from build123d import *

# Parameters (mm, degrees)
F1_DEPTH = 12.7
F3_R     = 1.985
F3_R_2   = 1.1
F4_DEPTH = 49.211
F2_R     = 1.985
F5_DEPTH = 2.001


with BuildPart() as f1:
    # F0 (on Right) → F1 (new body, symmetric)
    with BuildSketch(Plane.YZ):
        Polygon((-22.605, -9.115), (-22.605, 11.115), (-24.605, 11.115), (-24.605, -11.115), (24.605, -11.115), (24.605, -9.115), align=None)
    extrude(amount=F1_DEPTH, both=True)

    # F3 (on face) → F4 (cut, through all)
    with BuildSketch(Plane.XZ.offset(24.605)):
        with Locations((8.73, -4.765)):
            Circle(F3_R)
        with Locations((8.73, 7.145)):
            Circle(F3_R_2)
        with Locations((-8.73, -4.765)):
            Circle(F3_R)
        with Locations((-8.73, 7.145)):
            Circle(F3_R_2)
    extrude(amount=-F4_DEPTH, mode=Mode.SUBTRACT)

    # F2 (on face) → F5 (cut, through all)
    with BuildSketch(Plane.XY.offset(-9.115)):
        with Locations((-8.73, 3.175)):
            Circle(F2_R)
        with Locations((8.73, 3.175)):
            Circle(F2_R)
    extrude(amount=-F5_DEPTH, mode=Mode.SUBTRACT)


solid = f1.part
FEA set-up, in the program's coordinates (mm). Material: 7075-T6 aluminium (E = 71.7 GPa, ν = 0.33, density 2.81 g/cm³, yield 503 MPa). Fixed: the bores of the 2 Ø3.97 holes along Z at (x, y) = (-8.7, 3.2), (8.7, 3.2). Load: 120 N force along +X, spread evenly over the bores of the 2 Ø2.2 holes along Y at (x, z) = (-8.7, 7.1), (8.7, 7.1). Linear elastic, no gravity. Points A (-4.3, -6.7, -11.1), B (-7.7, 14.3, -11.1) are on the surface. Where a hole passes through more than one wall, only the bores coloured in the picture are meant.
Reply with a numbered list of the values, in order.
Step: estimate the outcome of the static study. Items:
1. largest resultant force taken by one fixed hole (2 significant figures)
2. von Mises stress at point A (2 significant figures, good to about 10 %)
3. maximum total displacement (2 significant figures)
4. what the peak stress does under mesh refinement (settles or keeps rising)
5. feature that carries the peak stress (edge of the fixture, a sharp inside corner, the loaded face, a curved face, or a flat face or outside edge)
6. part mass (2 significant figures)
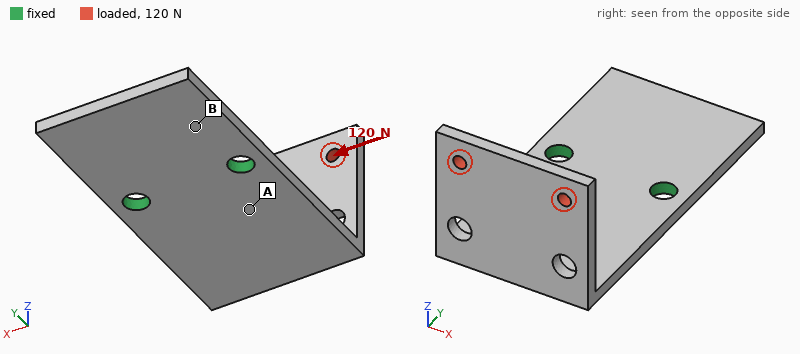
1. 210 N
2. 76 MPa
3. 0.50 mm
4. keeps rising
5. edge of the fixture
6. 9.6 g
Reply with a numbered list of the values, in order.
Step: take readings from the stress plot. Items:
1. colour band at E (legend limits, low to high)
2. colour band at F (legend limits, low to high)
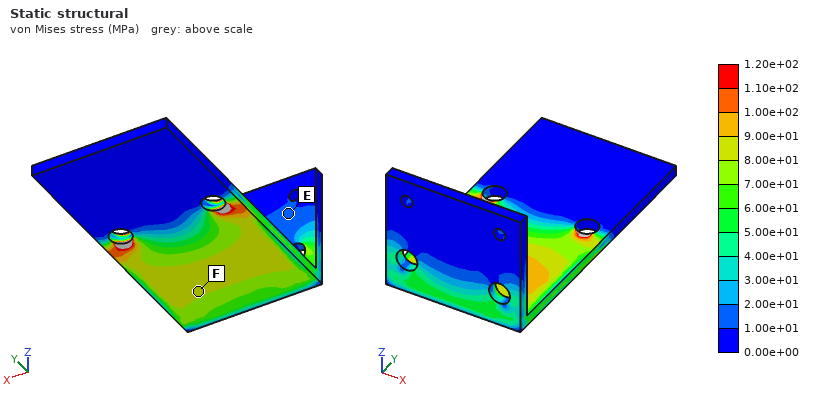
1. 1.00e+01 to 2.00e+01 MPa
2. 8.00e+01 to 9.00e+01 MPa
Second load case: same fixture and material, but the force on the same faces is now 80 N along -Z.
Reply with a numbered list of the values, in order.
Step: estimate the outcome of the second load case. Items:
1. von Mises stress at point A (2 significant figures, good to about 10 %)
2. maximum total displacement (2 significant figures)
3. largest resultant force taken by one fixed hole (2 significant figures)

1. 72 MPa
2. 0.60 mm
3. 40 N
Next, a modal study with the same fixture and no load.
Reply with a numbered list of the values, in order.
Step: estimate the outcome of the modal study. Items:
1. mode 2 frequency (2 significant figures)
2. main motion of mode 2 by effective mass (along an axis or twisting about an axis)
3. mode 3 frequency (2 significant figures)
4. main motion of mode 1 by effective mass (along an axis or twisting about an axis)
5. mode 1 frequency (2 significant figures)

1. 2000 Hz
2. along X
3. 2900 Hz
4. along Z
5. 1000 Hz
